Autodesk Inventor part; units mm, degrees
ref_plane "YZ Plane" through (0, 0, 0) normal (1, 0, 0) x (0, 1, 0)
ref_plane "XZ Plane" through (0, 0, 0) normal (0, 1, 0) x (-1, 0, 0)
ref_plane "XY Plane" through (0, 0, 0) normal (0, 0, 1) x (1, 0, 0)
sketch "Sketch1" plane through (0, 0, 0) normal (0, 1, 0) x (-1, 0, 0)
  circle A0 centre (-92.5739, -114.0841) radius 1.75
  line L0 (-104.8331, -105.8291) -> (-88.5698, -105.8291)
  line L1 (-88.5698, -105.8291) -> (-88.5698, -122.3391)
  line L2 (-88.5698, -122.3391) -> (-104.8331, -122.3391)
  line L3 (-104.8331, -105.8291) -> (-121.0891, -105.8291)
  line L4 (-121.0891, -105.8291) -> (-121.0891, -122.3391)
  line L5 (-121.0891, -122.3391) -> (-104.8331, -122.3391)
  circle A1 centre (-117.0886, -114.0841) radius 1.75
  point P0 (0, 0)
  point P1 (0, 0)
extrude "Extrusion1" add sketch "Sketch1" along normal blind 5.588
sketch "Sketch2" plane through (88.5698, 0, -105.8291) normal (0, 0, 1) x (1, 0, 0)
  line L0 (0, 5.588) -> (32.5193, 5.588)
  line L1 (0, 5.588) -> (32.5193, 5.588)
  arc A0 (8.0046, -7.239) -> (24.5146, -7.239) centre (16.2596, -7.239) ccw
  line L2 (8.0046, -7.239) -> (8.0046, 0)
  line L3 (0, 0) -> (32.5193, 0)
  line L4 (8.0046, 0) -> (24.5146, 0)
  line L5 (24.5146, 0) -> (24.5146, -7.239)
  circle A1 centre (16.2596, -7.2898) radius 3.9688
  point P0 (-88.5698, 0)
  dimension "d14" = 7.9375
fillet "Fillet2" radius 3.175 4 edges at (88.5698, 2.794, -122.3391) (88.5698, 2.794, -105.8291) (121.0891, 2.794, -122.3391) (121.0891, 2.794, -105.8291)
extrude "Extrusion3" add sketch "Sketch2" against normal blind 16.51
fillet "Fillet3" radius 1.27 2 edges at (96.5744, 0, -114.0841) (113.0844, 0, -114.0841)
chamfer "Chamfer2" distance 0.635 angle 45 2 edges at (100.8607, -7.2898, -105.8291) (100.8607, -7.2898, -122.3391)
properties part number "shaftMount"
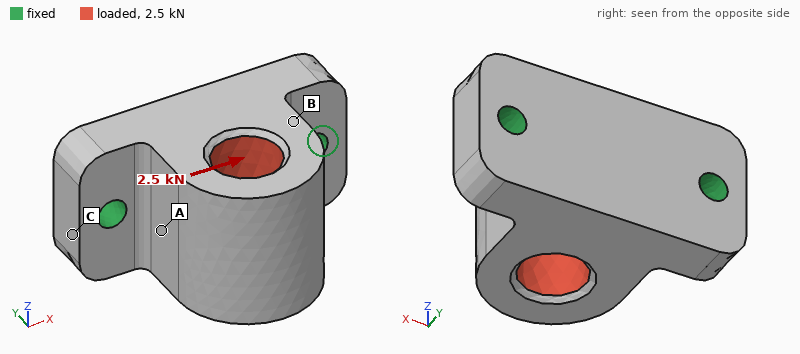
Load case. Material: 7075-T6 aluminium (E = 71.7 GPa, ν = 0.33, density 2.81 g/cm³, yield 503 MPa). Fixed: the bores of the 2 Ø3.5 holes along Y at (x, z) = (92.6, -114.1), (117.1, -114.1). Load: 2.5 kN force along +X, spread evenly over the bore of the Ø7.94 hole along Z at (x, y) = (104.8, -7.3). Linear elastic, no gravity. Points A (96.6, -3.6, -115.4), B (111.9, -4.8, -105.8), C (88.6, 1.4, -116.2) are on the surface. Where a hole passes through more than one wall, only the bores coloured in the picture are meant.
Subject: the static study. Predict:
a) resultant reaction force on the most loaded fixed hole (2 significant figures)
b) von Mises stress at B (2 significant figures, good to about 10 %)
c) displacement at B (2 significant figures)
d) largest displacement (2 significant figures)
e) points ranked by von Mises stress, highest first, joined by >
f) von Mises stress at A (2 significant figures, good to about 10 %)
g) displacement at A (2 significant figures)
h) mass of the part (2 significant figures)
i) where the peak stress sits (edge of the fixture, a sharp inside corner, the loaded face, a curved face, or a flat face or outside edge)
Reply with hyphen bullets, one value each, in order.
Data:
- 1.7 kN
- 21 MPa
- 8.5 µm
- 19 µm
- A > B > C
- 32 MPa
- 8.2 µm
- 16 g
- a curved face
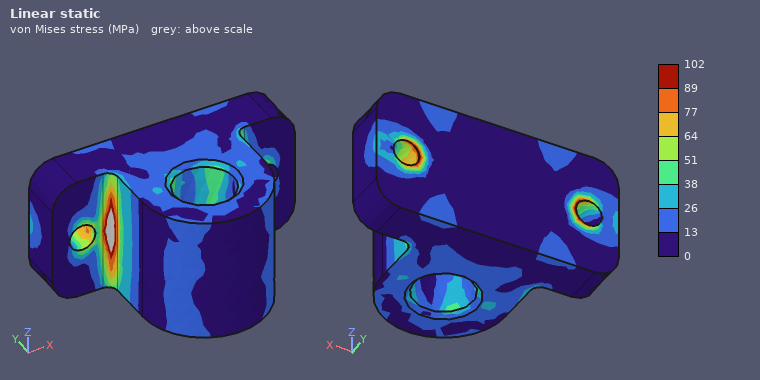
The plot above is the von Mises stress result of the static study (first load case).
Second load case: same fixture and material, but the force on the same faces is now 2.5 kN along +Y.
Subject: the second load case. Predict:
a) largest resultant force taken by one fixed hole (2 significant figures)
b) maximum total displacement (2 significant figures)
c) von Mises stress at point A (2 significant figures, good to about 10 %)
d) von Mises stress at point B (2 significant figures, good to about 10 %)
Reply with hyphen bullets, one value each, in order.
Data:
- 1.3 kN
- 8.2 µm
- 21 MPa
- 10 MPa
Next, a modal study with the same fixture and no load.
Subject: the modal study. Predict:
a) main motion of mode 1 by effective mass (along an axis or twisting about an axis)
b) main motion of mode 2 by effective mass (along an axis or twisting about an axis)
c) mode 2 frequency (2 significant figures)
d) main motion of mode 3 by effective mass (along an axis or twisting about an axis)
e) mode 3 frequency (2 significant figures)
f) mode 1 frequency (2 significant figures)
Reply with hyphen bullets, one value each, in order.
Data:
- along Z
- along X
- 23 kHz
- along Y
- 27 kHz
- 12 kHz
